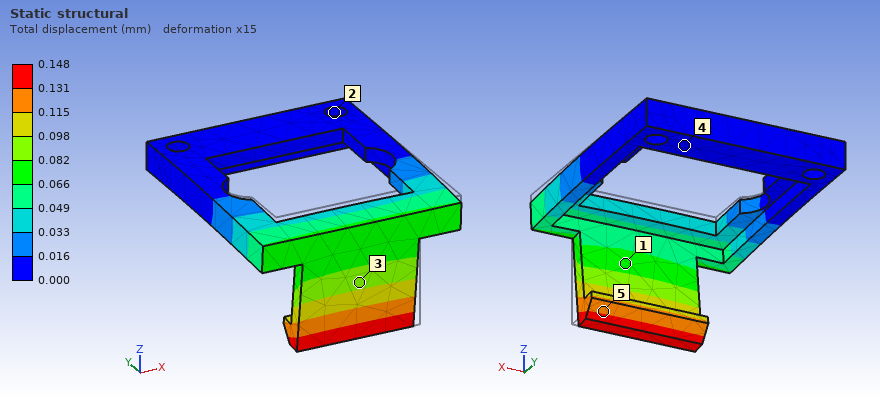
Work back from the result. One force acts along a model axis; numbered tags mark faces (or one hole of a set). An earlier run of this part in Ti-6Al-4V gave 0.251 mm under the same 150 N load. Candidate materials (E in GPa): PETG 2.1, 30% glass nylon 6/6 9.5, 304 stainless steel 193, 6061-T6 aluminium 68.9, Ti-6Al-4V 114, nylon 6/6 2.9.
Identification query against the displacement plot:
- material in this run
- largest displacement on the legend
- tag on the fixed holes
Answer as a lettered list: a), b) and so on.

a) 304 stainless steel
b) 0.148 mm
c) 2
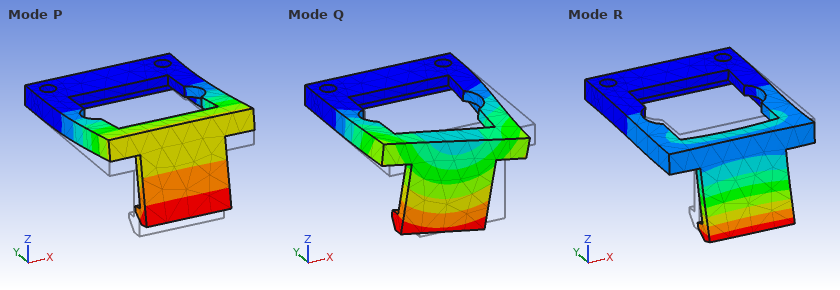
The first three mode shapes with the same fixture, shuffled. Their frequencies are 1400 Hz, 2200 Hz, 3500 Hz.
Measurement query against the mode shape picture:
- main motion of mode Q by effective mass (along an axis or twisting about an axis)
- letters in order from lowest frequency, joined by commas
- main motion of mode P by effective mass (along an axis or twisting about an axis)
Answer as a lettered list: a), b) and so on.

a) along X
b) P, Q, R
c) along Z
